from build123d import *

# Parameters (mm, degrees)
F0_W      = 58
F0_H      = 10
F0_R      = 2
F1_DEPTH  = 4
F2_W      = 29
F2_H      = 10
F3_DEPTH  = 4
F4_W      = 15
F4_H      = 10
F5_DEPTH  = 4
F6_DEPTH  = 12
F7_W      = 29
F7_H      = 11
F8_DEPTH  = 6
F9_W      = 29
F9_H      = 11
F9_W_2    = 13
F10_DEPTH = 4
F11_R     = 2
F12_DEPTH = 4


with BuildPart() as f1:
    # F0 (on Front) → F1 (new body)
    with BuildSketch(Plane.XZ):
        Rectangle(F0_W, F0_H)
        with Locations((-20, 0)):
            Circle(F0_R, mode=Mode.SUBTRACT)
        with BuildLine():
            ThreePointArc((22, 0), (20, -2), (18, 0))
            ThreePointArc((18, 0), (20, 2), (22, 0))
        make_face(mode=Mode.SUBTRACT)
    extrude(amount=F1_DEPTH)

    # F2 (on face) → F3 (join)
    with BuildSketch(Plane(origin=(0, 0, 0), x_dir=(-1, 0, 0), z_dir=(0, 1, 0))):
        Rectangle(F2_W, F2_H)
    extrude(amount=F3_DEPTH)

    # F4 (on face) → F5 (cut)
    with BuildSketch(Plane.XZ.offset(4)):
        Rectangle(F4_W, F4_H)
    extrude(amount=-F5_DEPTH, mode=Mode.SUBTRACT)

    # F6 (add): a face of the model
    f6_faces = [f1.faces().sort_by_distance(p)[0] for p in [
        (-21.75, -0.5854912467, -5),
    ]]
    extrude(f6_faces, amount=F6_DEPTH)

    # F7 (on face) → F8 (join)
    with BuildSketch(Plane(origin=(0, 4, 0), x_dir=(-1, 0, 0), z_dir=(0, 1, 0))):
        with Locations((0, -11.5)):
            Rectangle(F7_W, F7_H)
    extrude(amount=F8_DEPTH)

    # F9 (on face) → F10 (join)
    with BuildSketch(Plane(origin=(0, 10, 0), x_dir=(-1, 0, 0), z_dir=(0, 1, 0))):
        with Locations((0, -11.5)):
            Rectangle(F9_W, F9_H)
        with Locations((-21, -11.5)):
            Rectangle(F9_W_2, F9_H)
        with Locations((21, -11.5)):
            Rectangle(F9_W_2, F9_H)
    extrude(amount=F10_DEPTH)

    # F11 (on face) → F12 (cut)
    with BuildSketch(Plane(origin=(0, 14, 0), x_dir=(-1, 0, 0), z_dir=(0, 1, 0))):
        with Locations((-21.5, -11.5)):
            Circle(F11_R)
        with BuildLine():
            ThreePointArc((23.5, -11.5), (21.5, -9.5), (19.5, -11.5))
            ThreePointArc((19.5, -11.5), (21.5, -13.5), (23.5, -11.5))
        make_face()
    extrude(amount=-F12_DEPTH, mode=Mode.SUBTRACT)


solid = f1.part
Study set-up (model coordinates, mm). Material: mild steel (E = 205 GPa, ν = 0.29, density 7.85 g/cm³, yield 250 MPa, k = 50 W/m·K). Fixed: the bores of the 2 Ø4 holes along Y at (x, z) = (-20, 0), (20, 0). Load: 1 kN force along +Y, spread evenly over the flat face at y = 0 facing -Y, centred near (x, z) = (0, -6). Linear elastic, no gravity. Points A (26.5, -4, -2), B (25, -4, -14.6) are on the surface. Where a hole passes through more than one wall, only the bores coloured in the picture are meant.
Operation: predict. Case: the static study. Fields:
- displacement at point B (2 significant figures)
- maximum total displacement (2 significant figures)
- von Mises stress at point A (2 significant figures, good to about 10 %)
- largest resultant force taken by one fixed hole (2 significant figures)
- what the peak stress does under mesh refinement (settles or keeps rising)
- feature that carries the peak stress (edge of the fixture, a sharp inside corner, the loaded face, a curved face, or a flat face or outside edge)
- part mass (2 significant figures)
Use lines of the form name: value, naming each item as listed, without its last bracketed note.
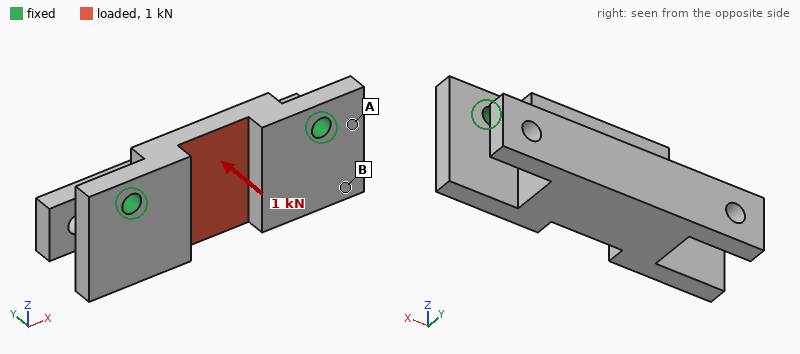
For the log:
displacement at point B: 6.0 µm
maximum total displacement: 15 µm
von Mises stress at point A: 20 MPa
largest resultant force taken by one fixed hole: 660 N
what the peak stress does under mesh refinement: keeps rising
feature that carries the peak stress: edge of the fixture
part mass: 82 g
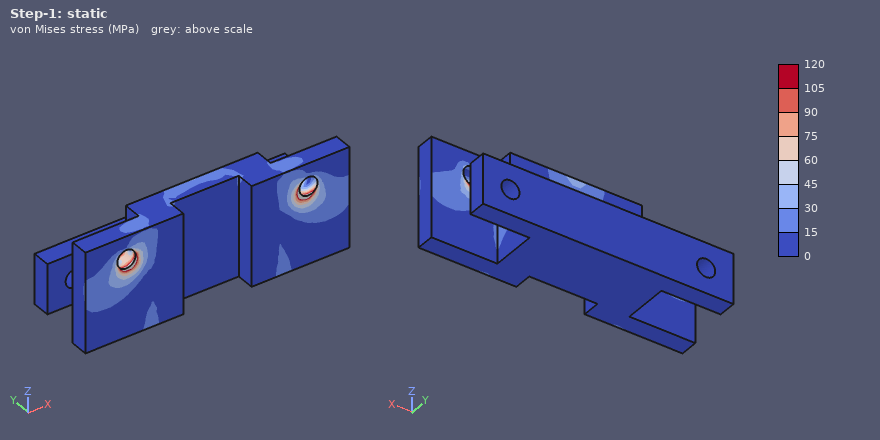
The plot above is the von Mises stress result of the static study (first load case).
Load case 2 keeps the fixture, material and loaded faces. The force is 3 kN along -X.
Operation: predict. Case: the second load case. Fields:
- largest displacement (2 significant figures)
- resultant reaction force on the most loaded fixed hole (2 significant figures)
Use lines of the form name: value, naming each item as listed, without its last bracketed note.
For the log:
largest displacement: 3.5 µm
resultant reaction force on the most loaded fixed hole: 1.6 kN
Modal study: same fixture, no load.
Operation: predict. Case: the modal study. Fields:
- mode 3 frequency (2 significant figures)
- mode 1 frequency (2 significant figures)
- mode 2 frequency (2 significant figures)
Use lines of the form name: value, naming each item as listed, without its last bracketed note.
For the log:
mode 3 frequency: 12 kHz
mode 1 frequency: 4100 Hz
mode 2 frequency: 9300 Hz
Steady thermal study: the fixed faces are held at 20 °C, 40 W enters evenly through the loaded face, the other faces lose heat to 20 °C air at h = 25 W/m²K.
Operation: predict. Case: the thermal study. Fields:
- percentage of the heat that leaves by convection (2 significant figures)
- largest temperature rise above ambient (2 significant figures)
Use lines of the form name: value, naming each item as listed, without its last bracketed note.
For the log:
percentage of the heat that leaves by convection: 13 %
largest temperature rise above ambient: 74 K
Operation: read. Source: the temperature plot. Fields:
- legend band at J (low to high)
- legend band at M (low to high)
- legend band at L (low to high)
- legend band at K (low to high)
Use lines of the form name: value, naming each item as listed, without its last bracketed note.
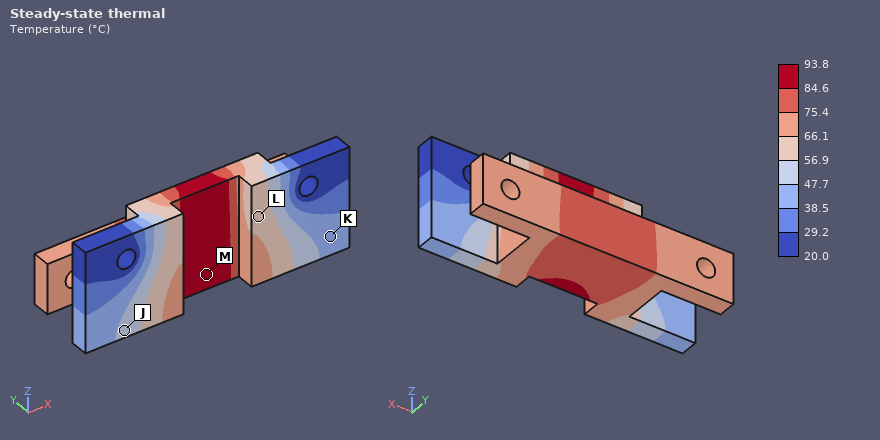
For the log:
legend band at J: 47.7 to 56.9 °C
legend band at M: 84.6 to 93.8 °C
legend band at L: 56.9 to 66.1 °C
legend band at K: 38.5 to 47.7 °C
